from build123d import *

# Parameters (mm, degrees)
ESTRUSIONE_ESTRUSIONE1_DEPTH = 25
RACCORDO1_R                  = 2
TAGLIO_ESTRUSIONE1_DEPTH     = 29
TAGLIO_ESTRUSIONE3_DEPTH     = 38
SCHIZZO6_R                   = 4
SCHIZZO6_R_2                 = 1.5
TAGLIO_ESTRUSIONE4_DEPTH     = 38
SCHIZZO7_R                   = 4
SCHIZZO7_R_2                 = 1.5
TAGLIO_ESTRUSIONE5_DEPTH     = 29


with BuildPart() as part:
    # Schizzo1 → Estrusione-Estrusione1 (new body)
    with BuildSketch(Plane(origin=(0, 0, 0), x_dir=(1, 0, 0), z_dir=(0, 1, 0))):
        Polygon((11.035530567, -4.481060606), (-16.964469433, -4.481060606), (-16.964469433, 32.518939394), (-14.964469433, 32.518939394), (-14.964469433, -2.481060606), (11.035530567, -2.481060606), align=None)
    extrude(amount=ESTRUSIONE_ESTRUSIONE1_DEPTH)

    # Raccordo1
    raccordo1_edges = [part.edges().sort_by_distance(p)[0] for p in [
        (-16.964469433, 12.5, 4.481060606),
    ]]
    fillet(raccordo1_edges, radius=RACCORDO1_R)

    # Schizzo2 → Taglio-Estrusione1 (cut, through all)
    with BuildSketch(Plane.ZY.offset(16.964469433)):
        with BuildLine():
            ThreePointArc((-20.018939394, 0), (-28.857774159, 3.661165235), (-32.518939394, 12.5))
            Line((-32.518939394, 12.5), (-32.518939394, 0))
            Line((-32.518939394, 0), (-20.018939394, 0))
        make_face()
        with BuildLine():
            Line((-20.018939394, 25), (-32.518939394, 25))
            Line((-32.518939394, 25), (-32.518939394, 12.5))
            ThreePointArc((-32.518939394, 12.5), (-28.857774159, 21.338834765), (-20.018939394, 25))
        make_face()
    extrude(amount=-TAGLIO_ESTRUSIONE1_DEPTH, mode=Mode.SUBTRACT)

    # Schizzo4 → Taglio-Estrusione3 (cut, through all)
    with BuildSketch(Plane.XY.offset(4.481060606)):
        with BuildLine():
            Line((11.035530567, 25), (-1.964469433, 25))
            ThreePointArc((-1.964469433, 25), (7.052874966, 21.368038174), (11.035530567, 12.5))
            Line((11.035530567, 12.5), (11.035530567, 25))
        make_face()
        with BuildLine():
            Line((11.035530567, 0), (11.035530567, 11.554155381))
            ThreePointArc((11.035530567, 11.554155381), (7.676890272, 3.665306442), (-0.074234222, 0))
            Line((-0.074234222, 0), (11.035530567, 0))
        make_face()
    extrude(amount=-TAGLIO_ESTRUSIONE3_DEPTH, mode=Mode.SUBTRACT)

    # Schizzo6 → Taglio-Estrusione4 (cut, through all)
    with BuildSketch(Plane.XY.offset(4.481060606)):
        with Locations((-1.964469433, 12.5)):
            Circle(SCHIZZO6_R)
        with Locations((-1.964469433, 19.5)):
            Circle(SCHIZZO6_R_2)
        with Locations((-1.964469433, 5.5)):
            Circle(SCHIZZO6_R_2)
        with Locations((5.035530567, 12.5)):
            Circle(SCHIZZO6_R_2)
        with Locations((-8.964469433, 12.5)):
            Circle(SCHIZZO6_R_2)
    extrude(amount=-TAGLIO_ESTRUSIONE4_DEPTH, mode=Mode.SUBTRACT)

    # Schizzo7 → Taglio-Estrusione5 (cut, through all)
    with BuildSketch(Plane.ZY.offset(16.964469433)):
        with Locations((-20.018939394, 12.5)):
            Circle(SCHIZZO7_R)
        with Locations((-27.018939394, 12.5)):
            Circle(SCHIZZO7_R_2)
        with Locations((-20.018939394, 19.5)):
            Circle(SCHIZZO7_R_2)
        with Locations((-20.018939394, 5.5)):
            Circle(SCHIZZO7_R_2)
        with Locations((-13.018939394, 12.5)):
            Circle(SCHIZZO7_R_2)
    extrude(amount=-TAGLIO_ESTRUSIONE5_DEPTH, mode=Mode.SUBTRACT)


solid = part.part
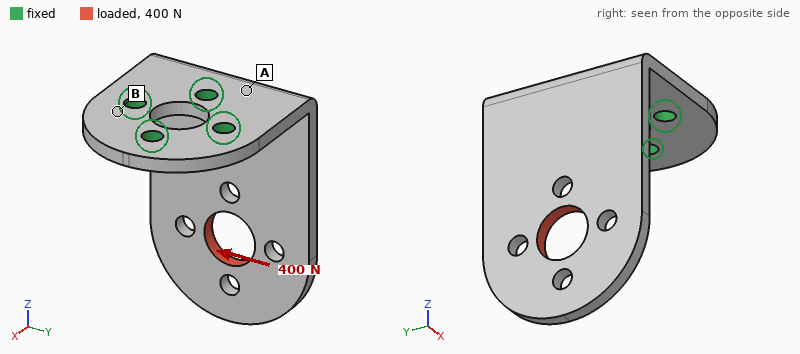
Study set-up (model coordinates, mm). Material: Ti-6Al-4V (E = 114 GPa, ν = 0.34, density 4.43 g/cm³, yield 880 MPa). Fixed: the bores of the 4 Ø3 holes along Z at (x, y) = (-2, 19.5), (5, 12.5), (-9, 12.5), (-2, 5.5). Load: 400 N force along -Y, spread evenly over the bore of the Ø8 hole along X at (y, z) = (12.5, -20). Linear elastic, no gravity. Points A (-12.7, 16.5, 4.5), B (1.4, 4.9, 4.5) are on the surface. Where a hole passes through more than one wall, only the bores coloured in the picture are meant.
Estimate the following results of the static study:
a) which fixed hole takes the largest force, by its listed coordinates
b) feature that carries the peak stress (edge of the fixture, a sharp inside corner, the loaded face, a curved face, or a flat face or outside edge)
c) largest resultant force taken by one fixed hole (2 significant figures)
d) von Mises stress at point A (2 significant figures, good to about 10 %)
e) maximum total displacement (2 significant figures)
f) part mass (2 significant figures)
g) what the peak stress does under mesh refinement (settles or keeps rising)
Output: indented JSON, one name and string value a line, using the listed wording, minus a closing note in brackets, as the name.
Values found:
{
  "which fixed hole takes the largest force, by its listed coordinates": "(-9, 12.5)",
  "feature that carries the peak stress": "edge of the fixture",
  "largest resultant force taken by one fixed hole": "370 N",
  "von Mises stress at point A": "200 MPa",
  "maximum total displacement": "0.61 mm",
  "part mass": "11 g",
  "what the peak stress does under mesh refinement": "keeps rising"
}
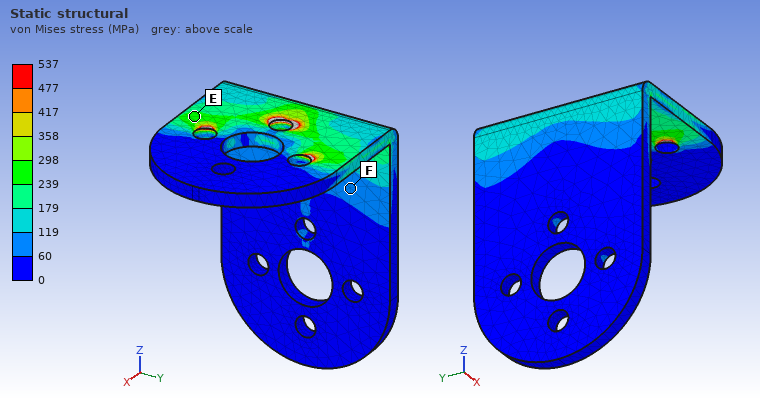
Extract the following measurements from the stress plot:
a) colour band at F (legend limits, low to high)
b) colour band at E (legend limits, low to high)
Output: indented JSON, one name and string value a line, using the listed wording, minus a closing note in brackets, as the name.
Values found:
{
  "colour band at F": "60 to 119 MPa",
  "colour band at E": "239 to 298 MPa"
}
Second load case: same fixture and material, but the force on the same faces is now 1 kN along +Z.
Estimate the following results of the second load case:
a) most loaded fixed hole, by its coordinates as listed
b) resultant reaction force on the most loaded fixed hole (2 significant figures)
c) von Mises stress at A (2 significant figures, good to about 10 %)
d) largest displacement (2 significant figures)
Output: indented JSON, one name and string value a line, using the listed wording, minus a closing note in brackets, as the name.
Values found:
{
  "most loaded fixed hole, by its coordinates as listed": "(-9, 12.5)",
  "resultant reaction force on the most loaded fixed hole": "1.2 kN",
  "von Mises stress at A": "210 MPa",
  "largest displacement": "0.51 mm"
}
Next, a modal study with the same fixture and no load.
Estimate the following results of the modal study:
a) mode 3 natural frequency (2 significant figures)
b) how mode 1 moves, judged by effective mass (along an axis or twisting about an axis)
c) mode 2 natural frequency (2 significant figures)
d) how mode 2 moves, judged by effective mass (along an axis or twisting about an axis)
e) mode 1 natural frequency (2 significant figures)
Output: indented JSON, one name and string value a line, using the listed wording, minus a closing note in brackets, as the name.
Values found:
{
  "mode 3 natural frequency": "4500 Hz",
  "how mode 1 moves, judged by effective mass": "along X",
  "mode 2 natural frequency": "2200 Hz",
  "how mode 2 moves, judged by effective mass": "along Y",
  "mode 1 natural frequency": "1200 Hz"
}
